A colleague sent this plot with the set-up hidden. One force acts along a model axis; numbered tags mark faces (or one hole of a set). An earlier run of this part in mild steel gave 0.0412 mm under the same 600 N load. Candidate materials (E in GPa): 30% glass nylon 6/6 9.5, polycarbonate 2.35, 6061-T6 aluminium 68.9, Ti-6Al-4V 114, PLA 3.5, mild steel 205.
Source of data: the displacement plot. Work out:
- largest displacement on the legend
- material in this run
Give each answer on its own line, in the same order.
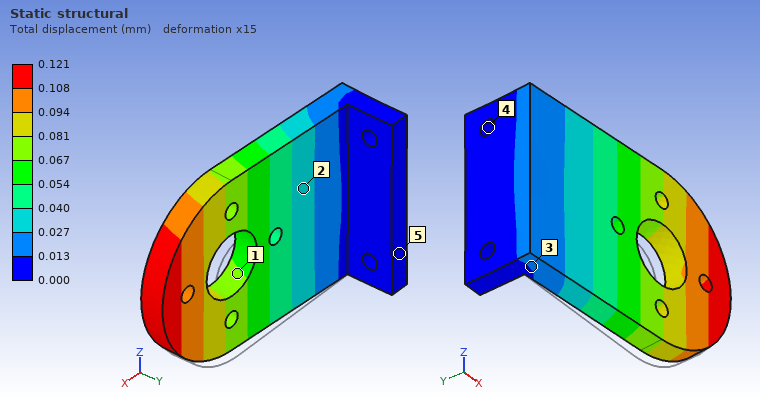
0.121 mm
6061-T6 aluminium
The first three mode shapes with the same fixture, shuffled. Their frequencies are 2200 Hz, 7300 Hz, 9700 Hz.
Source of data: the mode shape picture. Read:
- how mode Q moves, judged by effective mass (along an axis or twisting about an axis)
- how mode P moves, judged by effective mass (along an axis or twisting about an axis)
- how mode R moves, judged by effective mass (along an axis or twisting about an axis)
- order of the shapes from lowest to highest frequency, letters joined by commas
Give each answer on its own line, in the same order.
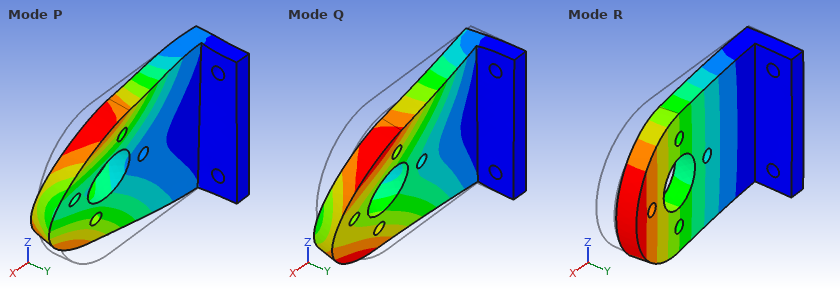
along Z
along Z
along Y
R, Q, P
